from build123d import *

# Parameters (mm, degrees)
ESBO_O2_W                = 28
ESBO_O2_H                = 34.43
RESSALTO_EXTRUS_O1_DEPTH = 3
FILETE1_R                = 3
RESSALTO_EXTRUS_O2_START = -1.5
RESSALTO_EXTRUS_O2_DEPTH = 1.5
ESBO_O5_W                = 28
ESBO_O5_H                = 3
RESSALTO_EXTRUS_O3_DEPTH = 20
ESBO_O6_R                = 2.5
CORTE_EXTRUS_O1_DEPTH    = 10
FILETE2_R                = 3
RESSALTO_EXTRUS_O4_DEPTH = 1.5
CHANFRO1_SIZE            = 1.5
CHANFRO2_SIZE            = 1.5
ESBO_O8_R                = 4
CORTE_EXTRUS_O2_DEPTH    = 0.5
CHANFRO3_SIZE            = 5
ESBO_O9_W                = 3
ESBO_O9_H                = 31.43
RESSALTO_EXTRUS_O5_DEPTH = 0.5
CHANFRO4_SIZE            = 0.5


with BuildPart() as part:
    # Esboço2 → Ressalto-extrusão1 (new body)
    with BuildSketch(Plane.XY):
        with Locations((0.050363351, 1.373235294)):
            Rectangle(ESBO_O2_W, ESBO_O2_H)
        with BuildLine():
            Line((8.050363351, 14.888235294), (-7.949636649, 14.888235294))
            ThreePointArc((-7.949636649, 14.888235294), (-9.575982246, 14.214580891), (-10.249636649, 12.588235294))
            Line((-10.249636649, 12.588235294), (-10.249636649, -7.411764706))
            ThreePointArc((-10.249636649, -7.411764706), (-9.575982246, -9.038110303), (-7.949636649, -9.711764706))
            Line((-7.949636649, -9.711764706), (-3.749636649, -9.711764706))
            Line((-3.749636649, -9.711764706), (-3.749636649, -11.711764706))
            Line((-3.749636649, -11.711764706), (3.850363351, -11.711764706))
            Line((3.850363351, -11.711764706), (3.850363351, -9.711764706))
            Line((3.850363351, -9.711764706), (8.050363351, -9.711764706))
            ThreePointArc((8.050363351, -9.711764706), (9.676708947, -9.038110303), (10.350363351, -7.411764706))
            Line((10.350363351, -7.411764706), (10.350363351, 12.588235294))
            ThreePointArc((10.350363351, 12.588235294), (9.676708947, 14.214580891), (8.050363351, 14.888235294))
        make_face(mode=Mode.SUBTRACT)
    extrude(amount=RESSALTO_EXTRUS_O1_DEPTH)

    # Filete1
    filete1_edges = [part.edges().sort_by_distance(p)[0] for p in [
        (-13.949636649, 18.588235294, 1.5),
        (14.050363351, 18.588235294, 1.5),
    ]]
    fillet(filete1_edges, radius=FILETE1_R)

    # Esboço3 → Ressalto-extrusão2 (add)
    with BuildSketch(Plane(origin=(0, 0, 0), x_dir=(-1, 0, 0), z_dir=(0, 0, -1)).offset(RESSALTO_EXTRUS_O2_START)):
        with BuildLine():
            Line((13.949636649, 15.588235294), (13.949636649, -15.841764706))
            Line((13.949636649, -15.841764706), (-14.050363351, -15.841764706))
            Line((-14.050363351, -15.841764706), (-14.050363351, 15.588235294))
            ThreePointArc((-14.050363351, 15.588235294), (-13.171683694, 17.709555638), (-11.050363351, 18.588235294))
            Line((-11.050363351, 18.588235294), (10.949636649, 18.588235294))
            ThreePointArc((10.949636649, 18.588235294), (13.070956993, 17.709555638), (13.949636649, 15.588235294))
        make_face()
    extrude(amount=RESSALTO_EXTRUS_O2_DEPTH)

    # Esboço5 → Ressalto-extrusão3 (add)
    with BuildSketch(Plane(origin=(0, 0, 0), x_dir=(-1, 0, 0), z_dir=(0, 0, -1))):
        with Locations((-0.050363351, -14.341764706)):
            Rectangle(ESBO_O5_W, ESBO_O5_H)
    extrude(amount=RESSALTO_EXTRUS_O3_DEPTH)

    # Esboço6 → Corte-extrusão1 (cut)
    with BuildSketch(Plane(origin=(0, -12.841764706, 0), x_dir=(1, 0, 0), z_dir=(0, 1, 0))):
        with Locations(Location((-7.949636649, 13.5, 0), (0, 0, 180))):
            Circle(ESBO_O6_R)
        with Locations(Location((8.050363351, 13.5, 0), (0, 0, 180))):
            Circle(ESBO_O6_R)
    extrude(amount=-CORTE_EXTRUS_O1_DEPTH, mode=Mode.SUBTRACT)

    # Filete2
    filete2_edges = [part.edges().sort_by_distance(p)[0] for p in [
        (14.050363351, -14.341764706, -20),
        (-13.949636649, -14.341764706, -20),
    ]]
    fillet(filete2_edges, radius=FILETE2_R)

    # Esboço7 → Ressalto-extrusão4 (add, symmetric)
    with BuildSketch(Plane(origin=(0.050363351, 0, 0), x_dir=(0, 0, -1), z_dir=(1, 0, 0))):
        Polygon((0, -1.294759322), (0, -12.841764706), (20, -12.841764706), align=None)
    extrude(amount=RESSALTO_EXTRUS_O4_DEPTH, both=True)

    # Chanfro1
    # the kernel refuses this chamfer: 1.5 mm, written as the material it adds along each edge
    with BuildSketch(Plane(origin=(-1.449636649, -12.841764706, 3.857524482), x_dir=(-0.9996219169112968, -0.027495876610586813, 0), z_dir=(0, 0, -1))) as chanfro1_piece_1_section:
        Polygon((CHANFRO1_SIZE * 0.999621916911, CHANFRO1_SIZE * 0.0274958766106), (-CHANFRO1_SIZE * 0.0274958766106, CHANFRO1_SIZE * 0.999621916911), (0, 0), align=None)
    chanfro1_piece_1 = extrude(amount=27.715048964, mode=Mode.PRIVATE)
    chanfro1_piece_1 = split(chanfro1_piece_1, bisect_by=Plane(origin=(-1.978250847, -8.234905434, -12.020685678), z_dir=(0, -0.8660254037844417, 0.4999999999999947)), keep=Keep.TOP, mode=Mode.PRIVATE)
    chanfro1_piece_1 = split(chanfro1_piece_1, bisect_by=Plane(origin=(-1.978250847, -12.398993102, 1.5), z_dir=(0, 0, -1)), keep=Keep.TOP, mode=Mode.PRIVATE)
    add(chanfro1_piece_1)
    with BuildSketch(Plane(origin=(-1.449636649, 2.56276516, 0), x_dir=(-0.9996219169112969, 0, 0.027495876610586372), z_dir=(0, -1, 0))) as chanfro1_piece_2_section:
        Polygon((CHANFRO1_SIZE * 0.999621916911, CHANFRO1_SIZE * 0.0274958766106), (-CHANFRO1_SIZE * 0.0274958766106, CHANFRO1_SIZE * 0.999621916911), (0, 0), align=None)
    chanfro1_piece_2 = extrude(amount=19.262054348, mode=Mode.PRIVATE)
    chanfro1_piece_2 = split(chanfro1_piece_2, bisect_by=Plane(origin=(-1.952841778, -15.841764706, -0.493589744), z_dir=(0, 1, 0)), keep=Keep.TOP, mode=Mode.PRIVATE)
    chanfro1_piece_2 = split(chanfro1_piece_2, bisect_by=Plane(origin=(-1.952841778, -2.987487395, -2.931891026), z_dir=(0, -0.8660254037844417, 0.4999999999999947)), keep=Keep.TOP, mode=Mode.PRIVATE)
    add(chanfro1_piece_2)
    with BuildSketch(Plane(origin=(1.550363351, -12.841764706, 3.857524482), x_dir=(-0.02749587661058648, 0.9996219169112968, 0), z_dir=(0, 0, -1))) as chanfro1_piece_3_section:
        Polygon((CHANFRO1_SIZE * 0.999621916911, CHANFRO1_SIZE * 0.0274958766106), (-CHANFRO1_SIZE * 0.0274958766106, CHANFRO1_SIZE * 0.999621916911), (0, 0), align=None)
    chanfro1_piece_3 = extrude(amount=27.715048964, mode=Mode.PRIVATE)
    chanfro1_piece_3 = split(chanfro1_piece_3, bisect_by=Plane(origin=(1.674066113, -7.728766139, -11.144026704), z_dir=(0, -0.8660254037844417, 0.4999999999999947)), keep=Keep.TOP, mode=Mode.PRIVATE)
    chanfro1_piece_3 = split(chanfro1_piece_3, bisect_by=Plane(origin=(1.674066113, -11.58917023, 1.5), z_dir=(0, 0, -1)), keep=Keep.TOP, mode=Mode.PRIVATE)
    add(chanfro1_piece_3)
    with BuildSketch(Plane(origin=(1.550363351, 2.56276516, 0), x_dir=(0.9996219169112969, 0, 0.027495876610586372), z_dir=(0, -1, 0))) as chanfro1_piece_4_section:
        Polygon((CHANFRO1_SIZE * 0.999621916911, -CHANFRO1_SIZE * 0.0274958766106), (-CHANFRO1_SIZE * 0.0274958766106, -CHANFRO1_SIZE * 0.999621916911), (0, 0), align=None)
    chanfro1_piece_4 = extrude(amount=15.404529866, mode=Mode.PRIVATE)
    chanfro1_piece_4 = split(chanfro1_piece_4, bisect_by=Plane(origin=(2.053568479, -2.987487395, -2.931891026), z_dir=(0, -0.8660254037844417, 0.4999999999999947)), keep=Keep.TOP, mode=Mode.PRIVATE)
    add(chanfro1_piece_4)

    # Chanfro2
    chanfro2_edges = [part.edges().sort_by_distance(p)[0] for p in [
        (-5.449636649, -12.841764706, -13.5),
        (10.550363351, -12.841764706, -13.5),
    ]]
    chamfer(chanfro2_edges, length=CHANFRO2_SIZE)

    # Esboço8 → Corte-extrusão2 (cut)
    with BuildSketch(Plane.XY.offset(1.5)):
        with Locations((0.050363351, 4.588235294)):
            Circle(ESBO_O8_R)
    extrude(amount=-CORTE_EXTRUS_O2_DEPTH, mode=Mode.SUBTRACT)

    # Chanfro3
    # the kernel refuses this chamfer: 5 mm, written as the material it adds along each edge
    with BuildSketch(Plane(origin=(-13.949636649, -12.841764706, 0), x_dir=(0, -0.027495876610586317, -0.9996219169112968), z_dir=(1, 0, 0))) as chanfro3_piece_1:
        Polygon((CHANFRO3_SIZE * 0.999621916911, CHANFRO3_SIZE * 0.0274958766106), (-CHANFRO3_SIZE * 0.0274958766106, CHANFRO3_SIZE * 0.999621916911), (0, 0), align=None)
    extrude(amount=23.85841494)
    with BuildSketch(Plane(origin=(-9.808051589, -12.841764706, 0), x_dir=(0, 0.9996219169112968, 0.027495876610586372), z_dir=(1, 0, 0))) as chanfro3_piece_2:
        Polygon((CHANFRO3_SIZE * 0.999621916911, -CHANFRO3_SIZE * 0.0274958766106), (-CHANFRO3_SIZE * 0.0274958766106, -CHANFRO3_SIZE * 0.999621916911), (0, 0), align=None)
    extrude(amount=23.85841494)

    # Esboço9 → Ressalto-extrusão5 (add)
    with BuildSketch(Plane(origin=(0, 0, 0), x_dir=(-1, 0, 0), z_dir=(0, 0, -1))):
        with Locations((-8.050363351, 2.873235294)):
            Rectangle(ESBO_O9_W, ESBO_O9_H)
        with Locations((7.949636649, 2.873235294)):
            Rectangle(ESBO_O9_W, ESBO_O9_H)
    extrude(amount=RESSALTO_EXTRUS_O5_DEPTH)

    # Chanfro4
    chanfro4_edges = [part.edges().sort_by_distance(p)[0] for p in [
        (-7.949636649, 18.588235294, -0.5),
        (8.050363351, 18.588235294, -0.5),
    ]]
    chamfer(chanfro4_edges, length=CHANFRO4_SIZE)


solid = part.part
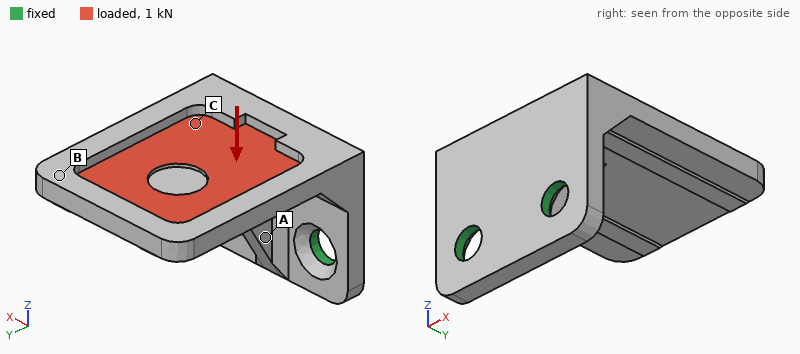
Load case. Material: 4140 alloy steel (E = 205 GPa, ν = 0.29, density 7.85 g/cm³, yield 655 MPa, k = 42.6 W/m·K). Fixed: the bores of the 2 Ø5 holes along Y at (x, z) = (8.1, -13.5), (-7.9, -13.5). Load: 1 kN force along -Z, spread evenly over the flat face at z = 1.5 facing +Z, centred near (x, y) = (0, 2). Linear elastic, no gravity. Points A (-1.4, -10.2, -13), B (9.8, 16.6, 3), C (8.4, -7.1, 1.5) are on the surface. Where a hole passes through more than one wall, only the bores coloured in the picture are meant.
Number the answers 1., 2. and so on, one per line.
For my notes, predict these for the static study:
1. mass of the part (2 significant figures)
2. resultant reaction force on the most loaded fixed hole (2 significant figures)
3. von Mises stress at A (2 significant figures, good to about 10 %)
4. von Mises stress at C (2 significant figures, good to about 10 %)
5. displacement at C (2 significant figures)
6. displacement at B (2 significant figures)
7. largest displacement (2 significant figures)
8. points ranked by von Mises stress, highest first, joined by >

1. 34 g
2. 520 N
3. 180 MPa
4. 110 MPa
5. 0.086 mm
6. 0.38 mm
7. 0.41 mm
8. A > C > B
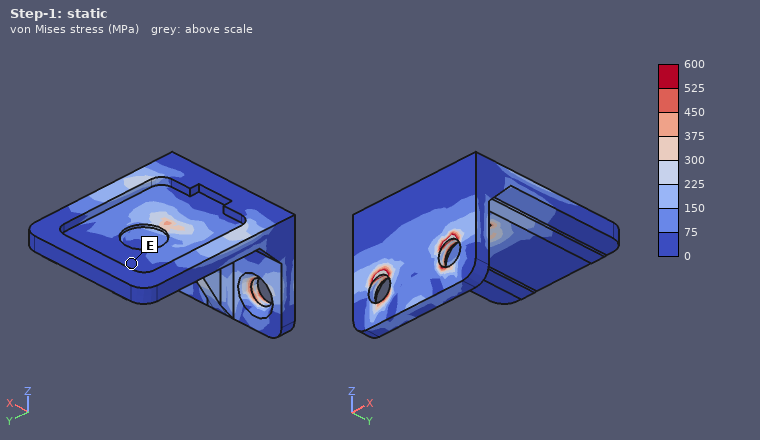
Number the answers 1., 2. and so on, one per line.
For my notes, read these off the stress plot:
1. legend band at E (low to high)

1. 0 to 75 MPa
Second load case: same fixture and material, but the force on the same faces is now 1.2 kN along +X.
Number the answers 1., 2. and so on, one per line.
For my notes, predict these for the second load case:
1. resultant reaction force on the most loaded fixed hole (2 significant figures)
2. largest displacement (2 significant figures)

1. 1.7 kN
2. 0.11 mm
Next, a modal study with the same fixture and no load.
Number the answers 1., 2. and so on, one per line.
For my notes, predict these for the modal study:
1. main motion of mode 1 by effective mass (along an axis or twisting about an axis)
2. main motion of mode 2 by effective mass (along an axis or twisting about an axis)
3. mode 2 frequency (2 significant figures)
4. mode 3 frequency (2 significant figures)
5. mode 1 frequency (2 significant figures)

1. along Z
2. along X
3. 4400 Hz
4. 5200 Hz
5. 2100 Hz
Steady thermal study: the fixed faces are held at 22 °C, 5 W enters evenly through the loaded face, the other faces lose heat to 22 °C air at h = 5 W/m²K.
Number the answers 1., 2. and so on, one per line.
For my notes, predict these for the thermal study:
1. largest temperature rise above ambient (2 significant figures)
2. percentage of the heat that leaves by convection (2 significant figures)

1. 37 K
2. 6.0 %
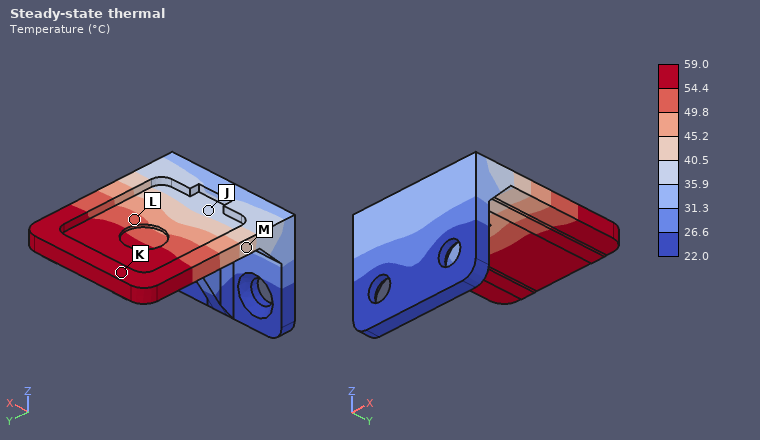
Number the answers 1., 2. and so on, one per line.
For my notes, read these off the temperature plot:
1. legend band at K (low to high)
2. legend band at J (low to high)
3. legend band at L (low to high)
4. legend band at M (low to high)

1. 54.4 to 59.0 °C
2. 35.9 to 40.5 °C
3. 49.8 to 54.4 °C
4. 40.5 to 45.2 °C
